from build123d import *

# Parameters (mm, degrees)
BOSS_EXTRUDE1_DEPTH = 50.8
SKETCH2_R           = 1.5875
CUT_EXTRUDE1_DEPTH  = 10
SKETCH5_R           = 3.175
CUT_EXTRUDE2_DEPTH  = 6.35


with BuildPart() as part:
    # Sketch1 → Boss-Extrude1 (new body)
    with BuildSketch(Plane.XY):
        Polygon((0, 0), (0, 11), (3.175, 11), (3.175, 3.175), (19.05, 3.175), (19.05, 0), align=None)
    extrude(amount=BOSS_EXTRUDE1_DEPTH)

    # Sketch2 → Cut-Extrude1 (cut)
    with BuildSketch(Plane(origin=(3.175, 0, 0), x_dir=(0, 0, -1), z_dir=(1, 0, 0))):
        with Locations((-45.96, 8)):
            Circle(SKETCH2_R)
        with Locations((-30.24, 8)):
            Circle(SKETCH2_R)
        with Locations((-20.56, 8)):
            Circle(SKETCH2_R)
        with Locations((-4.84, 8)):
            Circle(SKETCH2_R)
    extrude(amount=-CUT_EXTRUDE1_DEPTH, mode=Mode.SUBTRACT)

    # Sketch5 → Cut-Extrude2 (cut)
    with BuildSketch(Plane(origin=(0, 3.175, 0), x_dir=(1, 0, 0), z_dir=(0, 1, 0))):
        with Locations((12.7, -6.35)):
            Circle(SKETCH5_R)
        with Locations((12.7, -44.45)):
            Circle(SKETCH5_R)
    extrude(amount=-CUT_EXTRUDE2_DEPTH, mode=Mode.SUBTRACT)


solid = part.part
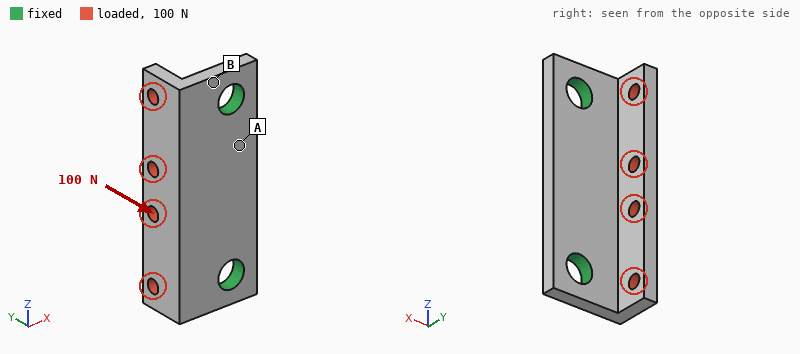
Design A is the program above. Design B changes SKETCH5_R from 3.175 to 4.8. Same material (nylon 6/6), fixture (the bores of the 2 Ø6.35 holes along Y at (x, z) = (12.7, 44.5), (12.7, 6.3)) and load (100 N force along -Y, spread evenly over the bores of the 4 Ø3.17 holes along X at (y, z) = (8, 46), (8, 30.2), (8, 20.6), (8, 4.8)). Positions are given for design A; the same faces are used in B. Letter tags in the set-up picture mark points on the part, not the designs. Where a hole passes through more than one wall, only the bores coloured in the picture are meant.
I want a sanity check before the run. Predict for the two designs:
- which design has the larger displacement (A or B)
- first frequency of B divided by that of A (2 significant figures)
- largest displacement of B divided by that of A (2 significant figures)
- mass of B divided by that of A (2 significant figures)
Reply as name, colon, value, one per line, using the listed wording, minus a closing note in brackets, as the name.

which design has the larger displacement: A
first frequency of B divided by that of A: 1.3
largest displacement of B divided by that of A: 0.62
mass of B divided by that of A: 0.94
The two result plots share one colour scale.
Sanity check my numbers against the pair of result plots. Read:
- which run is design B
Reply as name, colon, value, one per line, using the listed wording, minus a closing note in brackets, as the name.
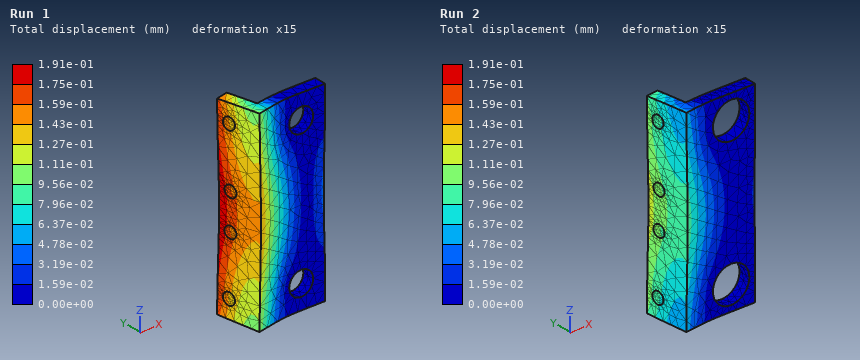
which run is design B: Run 2
